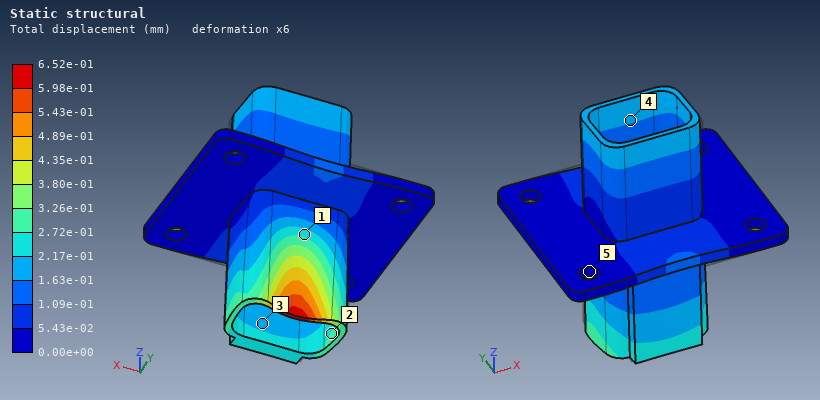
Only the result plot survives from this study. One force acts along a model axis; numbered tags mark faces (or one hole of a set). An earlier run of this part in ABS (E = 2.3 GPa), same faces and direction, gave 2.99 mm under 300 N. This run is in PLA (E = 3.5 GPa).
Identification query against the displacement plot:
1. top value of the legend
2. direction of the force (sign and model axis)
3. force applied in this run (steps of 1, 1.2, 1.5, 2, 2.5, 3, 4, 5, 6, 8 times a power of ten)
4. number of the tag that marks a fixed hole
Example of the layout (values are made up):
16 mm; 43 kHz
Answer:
6.52e-01 mm; -Y; 100 N; 5
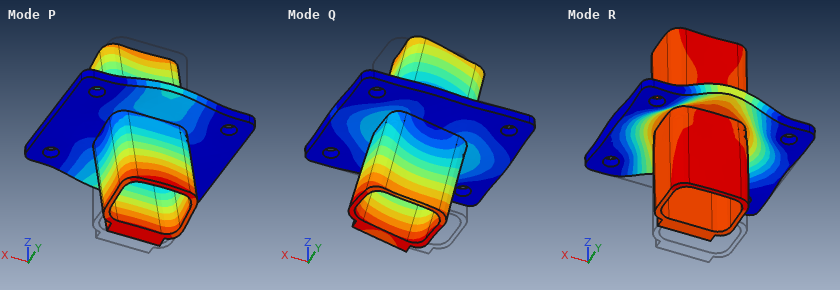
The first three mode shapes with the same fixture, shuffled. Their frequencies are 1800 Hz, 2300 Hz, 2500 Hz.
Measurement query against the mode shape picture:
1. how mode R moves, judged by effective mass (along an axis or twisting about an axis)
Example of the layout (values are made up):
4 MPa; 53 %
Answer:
along Z
